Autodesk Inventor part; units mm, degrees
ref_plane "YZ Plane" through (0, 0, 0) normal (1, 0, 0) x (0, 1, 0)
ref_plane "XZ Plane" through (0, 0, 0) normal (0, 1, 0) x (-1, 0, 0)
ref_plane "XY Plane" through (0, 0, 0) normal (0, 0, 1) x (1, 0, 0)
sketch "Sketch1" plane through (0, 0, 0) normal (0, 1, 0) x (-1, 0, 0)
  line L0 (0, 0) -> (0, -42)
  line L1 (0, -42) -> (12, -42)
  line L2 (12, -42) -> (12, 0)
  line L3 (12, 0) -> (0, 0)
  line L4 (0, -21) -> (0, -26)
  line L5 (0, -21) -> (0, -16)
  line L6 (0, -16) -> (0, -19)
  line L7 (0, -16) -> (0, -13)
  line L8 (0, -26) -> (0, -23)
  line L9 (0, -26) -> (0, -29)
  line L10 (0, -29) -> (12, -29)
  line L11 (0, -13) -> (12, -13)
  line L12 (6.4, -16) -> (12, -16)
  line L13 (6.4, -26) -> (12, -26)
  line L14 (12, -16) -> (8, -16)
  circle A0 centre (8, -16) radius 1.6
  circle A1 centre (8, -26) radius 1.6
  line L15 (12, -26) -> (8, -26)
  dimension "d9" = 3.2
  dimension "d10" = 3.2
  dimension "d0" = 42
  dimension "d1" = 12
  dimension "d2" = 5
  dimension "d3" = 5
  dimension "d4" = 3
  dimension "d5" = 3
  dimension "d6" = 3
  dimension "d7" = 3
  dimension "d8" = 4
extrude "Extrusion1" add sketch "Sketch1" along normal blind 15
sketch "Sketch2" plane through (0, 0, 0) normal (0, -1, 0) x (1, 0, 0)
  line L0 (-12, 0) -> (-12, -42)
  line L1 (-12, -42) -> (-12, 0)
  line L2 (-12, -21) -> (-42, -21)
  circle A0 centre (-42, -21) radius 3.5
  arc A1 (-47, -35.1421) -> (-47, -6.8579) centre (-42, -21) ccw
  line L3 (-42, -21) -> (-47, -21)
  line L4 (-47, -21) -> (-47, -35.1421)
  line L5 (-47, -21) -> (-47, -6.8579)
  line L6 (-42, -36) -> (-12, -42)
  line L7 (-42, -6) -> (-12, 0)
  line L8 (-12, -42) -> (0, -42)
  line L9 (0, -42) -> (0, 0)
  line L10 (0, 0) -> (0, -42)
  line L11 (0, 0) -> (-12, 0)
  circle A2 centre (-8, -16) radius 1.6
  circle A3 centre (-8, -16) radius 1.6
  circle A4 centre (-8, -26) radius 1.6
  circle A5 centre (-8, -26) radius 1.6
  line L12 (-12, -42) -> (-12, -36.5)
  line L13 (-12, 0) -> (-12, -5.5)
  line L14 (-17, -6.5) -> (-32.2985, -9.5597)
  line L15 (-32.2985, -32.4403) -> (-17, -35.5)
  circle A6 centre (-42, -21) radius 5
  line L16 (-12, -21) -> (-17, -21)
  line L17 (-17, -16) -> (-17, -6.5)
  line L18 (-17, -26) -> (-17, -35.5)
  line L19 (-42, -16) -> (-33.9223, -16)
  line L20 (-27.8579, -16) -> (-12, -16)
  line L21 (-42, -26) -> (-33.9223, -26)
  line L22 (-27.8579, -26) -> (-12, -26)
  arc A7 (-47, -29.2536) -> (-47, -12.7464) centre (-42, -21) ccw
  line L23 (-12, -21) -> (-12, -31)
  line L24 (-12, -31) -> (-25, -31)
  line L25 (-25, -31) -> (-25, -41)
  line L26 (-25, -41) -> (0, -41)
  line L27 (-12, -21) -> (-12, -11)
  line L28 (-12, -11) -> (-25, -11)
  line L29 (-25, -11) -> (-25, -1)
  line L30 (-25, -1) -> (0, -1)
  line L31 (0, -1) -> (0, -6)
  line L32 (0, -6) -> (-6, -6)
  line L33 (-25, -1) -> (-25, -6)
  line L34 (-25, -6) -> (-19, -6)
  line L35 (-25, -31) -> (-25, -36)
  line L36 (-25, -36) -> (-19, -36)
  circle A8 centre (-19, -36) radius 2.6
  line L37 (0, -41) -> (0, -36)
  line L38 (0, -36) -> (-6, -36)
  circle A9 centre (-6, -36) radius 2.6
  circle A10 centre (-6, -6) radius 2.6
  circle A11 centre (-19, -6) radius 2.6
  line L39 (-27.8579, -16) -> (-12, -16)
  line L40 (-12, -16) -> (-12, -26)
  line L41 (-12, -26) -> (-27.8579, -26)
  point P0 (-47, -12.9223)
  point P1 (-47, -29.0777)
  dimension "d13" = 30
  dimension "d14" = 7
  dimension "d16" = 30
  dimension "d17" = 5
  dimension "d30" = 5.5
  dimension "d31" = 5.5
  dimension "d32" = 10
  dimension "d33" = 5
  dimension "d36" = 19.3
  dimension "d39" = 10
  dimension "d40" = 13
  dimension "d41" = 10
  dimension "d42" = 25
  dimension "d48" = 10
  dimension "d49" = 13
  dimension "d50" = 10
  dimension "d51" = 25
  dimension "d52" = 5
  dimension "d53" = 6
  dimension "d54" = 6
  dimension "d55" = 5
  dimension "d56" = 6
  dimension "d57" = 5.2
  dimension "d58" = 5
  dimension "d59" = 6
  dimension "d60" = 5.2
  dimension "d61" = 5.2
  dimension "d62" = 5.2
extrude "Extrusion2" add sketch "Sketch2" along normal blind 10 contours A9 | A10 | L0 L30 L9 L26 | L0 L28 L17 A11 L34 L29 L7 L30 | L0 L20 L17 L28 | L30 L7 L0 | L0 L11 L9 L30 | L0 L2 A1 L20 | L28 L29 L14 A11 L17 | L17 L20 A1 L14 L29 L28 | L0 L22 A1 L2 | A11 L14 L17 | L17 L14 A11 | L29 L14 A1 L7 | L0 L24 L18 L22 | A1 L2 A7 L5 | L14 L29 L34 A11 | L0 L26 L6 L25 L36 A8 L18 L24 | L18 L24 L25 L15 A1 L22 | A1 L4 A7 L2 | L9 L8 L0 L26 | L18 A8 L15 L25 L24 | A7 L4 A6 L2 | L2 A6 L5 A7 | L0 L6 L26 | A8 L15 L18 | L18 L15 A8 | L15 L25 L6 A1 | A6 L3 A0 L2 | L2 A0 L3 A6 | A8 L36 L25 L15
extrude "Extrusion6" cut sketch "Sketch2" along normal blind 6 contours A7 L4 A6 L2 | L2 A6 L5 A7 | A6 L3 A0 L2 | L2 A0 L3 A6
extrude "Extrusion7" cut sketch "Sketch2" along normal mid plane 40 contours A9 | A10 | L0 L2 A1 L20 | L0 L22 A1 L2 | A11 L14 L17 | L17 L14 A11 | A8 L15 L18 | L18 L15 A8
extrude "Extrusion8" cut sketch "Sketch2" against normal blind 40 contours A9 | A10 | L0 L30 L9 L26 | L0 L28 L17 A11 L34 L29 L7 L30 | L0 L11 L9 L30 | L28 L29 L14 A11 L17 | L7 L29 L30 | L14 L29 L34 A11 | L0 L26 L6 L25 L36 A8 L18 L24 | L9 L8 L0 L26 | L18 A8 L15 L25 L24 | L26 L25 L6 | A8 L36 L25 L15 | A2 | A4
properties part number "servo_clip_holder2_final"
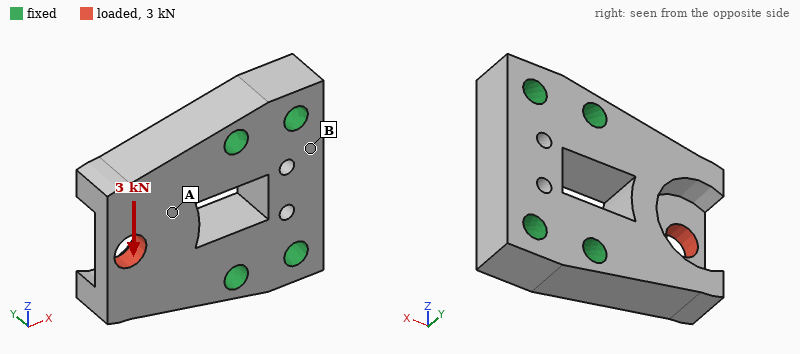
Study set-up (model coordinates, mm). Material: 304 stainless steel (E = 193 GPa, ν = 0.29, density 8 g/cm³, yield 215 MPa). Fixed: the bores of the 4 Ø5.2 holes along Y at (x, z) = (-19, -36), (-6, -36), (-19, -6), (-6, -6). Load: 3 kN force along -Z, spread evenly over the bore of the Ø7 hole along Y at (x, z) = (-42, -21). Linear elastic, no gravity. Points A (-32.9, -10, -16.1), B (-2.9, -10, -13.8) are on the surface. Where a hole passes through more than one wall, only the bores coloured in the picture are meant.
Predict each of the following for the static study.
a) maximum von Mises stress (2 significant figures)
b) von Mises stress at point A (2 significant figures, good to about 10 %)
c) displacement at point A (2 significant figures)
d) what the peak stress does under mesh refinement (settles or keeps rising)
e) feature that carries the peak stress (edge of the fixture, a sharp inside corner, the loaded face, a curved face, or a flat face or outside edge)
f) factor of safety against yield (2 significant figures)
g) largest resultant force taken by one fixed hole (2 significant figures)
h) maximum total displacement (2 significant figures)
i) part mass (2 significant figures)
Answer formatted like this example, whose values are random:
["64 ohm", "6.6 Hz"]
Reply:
["130 MPa", "34 MPa", "3.9 µm", "settles", "the loaded face", "1.7", "2.6 kN", "11 µm", "110 g"]
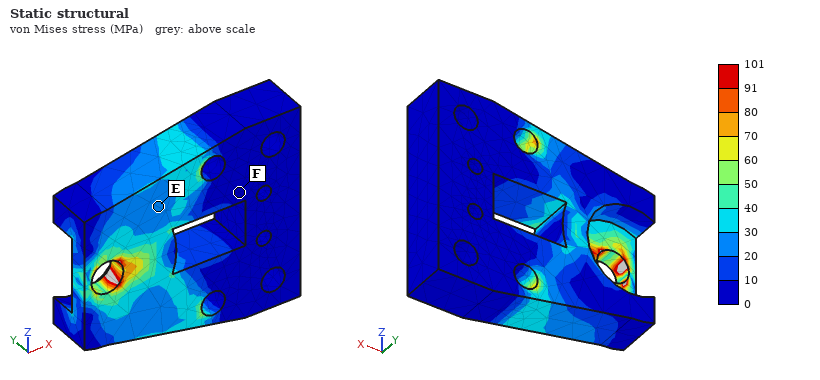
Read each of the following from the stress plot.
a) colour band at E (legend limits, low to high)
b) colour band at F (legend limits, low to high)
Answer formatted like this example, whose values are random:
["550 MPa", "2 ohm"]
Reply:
["20 to 30 MPa", "0 to 10 MPa"]
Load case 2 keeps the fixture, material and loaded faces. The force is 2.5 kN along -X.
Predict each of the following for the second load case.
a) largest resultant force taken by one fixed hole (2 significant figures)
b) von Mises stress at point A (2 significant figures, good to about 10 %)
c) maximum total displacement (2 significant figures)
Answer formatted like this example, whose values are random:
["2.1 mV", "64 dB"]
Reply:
["1.1 kN", "35 MPa", "10 µm"]
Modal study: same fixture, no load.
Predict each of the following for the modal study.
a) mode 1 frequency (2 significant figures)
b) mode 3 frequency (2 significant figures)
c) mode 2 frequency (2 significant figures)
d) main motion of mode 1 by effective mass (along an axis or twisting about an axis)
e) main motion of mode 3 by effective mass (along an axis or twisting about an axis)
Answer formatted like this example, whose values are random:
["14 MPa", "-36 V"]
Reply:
["11 kHz", "22 kHz", "16 kHz", "along Y", "along Z"]
